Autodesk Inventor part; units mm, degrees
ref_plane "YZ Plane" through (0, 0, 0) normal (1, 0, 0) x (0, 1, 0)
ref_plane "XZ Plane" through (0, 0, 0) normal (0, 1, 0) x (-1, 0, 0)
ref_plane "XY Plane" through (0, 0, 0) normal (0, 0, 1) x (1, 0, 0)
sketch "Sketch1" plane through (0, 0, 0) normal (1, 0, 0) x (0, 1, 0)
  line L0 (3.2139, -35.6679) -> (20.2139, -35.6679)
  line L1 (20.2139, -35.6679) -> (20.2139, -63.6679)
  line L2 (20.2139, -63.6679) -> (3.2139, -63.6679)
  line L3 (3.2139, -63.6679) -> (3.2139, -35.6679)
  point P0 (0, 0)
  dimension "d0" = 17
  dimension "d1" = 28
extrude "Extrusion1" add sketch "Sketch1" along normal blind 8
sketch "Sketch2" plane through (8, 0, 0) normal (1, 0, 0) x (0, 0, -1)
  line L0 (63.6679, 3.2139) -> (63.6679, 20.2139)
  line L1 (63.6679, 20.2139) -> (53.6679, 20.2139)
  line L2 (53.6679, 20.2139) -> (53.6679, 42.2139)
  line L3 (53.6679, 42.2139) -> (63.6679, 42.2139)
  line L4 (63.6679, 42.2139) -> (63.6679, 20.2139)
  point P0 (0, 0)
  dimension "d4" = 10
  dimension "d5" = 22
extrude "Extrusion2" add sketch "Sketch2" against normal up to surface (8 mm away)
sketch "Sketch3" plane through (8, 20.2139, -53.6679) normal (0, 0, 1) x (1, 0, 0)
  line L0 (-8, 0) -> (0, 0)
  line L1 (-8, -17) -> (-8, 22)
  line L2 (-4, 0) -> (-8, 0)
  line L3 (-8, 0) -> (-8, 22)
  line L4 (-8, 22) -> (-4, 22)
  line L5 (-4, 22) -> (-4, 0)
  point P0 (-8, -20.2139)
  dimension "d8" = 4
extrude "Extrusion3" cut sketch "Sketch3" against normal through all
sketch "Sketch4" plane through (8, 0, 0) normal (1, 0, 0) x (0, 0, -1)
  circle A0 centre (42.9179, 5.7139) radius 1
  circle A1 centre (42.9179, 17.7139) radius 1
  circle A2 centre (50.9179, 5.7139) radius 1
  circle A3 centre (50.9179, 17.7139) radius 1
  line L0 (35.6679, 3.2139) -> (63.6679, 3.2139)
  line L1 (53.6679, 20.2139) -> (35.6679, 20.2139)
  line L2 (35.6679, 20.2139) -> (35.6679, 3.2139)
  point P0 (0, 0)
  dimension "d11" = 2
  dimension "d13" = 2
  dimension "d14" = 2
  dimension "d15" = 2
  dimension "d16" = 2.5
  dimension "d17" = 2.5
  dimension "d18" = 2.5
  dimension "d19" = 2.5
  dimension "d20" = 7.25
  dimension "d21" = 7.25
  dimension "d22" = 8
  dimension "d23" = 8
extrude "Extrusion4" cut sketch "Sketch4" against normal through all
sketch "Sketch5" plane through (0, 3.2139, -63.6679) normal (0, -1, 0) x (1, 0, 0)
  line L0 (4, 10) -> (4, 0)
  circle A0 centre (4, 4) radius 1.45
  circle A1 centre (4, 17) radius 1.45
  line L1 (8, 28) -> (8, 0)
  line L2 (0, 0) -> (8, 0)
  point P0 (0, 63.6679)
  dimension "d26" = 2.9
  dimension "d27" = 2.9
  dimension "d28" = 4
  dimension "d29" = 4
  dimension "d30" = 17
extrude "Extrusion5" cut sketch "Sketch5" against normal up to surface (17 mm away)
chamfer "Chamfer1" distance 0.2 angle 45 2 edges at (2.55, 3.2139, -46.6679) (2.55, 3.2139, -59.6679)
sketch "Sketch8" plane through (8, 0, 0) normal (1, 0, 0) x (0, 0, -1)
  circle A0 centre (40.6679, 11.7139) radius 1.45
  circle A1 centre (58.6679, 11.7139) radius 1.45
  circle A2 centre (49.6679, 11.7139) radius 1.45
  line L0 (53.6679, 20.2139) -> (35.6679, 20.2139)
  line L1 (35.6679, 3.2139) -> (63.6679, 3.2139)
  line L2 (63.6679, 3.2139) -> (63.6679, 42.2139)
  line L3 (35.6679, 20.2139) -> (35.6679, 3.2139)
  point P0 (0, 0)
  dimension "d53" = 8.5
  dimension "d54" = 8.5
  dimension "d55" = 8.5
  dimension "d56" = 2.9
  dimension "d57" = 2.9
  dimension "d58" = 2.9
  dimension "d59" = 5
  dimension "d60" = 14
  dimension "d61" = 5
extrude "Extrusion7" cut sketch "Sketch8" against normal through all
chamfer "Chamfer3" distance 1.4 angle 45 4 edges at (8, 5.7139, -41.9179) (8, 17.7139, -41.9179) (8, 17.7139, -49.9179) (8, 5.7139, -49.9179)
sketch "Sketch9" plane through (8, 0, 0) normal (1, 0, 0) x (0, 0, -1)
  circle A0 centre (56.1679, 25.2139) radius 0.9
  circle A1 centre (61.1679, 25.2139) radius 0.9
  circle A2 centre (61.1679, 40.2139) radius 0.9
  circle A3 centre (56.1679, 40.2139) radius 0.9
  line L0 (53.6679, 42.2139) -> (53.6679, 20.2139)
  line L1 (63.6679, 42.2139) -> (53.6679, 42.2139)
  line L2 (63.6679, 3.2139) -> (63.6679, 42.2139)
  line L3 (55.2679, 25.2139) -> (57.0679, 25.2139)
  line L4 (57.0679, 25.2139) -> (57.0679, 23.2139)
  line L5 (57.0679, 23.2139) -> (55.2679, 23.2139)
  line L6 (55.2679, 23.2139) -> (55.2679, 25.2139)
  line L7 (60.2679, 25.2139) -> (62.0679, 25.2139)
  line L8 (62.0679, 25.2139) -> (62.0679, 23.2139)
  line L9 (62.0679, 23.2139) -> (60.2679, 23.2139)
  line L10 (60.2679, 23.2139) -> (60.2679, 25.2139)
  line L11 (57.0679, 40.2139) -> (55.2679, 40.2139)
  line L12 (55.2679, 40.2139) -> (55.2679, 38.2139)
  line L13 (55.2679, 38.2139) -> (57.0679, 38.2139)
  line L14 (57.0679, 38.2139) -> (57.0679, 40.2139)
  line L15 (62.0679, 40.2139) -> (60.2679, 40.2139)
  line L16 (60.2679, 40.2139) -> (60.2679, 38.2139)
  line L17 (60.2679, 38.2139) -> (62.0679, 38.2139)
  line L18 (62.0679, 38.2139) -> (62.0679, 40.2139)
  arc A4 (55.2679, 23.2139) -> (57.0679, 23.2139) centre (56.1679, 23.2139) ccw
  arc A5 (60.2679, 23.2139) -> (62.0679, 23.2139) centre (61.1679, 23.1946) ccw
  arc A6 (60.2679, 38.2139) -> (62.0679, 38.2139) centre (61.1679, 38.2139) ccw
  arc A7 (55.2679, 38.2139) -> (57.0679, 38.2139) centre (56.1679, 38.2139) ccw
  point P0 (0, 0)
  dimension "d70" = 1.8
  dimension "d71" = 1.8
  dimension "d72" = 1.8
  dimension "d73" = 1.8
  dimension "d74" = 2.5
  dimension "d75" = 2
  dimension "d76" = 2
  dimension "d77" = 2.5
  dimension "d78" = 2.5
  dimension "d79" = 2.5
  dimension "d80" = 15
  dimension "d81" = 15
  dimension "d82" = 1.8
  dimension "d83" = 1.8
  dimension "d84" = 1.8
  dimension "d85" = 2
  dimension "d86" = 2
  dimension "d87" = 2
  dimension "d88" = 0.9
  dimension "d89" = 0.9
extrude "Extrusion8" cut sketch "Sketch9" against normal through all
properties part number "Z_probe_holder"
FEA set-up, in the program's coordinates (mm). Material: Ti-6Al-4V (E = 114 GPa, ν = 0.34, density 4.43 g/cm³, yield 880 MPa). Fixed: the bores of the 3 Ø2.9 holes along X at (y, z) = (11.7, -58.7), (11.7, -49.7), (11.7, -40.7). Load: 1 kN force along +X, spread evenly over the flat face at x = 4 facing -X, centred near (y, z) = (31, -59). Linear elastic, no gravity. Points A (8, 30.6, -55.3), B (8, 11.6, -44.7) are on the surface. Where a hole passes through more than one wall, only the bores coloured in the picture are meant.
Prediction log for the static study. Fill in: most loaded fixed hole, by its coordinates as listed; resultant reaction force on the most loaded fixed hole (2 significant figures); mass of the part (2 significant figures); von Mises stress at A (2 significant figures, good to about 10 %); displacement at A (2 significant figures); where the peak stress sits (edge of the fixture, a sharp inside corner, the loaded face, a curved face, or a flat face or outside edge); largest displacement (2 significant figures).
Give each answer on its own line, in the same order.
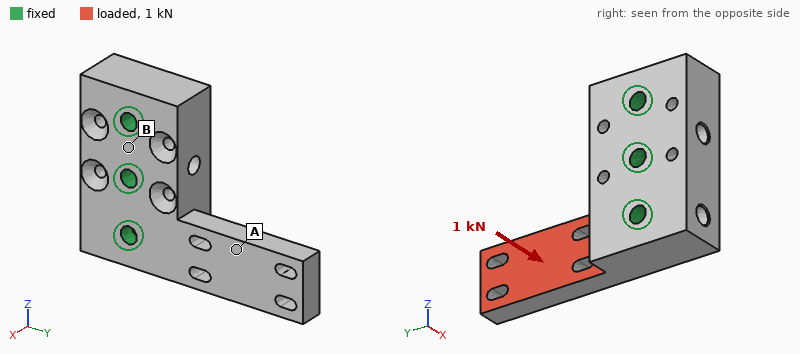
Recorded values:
(11.7, -58.7)
710 N
18 g
110 MPa
0.17 mm
the loaded face
0.43 mm
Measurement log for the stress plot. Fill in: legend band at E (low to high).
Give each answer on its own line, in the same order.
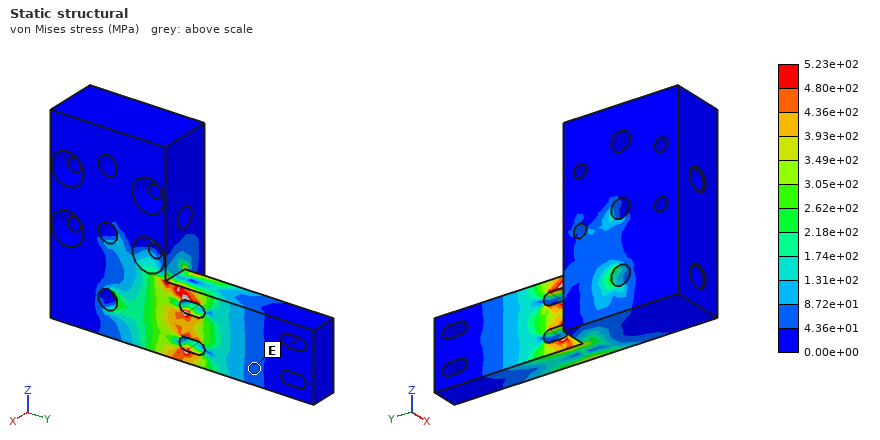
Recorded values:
4.36e+01 to 8.72e+01 MPa
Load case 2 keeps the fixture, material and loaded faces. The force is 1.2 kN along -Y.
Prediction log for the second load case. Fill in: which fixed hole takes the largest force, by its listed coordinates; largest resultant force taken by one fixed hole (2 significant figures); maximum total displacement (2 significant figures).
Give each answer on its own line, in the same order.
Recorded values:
(11.7, -58.7)
1.1 kN
0.10 mm
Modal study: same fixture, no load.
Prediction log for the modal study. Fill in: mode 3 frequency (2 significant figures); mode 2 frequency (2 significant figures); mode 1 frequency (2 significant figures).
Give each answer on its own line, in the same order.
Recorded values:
20 kHz
11 kHz
5200 Hz
